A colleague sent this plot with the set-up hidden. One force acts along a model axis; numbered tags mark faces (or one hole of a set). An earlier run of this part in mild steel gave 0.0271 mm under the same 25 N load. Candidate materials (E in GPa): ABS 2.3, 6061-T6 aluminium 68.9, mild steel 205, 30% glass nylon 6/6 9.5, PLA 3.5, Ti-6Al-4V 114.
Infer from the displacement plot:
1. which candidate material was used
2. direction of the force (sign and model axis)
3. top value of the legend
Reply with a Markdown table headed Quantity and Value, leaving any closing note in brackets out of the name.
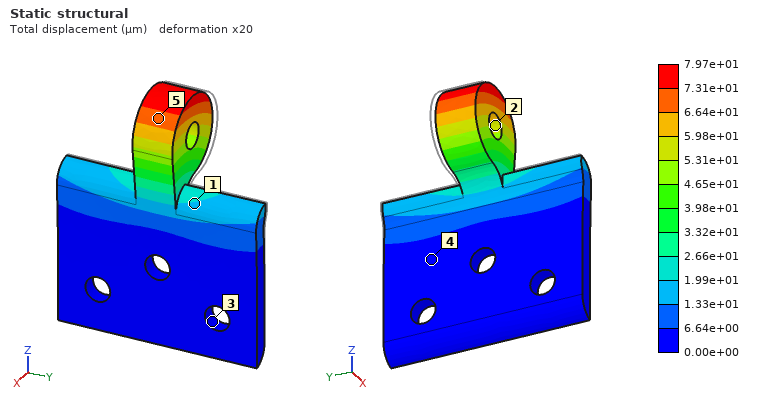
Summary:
| Quantity | Value |
|---|---|
| which candidate material was used | 6061-T6 aluminium |
| direction of the force | +X |
| top value of the legend | 7.97e+01 µm |
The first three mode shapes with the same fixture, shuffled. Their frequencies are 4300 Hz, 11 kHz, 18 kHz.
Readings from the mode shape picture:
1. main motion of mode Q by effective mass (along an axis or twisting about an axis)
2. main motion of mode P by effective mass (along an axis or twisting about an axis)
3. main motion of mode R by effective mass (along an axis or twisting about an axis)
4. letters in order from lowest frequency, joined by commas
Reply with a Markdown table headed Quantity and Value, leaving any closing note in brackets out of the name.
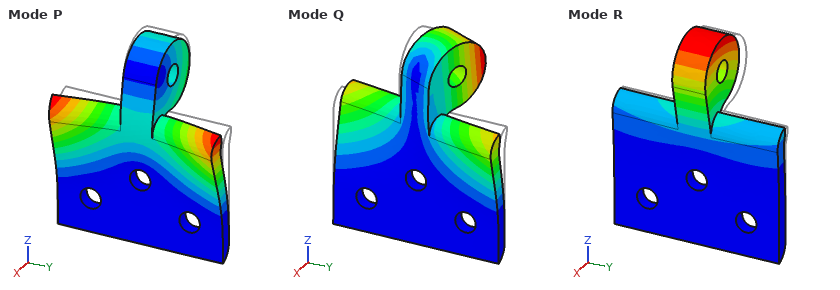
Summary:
| Quantity | Value |
|---|---|
| main motion of mode Q by effective mass | along Y |
| main motion of mode P by effective mass | along X |
| main motion of mode R by effective mass | along X |
| letters in order from lowest frequency, joined by commas | R, Q, P |
